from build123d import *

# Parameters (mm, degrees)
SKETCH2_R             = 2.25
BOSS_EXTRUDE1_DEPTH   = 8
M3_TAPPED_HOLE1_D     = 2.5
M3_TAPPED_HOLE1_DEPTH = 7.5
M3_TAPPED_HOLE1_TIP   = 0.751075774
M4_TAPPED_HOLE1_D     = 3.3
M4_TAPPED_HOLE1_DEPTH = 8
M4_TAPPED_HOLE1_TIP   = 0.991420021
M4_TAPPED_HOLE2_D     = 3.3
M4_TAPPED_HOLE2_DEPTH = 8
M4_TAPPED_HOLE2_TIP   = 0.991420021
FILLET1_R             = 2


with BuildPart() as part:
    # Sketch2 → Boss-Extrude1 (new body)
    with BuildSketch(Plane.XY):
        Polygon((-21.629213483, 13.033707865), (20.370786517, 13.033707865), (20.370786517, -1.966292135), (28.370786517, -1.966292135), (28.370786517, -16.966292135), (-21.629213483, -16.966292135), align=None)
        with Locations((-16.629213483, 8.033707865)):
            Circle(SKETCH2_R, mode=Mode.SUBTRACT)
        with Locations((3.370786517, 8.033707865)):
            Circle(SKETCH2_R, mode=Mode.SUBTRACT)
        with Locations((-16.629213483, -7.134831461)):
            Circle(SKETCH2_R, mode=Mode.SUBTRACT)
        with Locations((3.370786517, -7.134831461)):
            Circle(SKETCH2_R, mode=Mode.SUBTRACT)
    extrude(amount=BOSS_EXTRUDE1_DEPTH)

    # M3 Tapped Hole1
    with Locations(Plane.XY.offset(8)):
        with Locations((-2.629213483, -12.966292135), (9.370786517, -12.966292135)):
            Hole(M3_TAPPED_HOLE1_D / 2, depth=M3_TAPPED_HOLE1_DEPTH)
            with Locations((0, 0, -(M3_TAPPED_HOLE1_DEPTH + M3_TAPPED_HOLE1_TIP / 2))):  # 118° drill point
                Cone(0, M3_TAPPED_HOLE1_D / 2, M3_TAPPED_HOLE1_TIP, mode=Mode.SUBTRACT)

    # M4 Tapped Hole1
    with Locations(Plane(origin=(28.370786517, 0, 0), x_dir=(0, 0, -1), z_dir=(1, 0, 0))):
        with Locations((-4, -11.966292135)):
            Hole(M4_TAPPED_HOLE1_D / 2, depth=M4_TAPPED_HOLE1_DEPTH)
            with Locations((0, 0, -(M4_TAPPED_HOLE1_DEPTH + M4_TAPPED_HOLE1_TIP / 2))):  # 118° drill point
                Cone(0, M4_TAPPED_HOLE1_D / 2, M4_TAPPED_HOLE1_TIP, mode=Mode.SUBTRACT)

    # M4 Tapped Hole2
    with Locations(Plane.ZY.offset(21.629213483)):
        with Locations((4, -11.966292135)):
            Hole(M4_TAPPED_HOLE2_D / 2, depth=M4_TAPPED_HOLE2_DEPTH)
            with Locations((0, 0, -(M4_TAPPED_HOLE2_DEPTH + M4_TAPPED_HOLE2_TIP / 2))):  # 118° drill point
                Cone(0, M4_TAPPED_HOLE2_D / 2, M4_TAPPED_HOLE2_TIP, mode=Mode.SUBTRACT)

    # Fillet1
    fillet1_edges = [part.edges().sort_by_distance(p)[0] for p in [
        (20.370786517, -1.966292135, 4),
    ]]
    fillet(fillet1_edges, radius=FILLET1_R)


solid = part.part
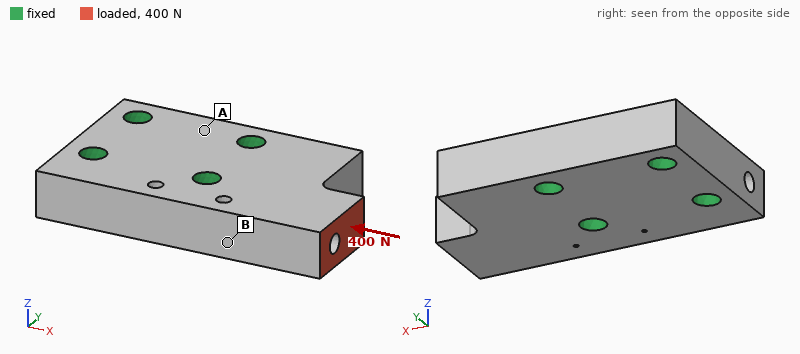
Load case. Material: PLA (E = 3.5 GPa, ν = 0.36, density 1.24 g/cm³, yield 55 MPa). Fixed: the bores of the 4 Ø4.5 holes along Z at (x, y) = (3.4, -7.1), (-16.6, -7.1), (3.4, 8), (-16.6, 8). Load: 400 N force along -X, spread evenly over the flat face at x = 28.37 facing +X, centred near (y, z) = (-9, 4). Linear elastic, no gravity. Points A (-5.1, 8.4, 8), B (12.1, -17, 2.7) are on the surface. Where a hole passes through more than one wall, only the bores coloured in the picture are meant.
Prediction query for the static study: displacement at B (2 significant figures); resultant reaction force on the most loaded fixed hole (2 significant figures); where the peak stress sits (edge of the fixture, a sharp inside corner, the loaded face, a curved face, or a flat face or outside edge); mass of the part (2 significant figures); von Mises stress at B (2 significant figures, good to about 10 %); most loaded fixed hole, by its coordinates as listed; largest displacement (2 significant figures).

19 µm
340 N
a curved face
13 g
4.0 MPa
(3.4, -7.1)
42 µm
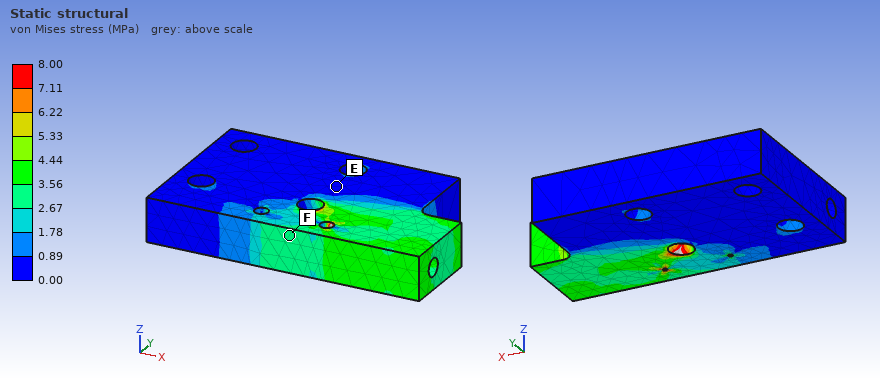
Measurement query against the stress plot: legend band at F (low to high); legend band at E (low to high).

2.67 to 3.56 MPa
0.00 to 0.89 MPa
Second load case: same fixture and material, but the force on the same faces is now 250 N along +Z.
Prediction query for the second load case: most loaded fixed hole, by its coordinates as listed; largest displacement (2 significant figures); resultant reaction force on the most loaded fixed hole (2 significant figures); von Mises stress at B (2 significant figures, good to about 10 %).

(3.4, -7.1)
0.47 mm
280 N
7.3 MPa
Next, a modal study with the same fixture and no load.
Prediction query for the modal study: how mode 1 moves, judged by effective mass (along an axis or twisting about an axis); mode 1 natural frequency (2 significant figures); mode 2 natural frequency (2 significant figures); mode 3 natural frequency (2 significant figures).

along Z
3900 Hz
8000 Hz
8200 Hz
